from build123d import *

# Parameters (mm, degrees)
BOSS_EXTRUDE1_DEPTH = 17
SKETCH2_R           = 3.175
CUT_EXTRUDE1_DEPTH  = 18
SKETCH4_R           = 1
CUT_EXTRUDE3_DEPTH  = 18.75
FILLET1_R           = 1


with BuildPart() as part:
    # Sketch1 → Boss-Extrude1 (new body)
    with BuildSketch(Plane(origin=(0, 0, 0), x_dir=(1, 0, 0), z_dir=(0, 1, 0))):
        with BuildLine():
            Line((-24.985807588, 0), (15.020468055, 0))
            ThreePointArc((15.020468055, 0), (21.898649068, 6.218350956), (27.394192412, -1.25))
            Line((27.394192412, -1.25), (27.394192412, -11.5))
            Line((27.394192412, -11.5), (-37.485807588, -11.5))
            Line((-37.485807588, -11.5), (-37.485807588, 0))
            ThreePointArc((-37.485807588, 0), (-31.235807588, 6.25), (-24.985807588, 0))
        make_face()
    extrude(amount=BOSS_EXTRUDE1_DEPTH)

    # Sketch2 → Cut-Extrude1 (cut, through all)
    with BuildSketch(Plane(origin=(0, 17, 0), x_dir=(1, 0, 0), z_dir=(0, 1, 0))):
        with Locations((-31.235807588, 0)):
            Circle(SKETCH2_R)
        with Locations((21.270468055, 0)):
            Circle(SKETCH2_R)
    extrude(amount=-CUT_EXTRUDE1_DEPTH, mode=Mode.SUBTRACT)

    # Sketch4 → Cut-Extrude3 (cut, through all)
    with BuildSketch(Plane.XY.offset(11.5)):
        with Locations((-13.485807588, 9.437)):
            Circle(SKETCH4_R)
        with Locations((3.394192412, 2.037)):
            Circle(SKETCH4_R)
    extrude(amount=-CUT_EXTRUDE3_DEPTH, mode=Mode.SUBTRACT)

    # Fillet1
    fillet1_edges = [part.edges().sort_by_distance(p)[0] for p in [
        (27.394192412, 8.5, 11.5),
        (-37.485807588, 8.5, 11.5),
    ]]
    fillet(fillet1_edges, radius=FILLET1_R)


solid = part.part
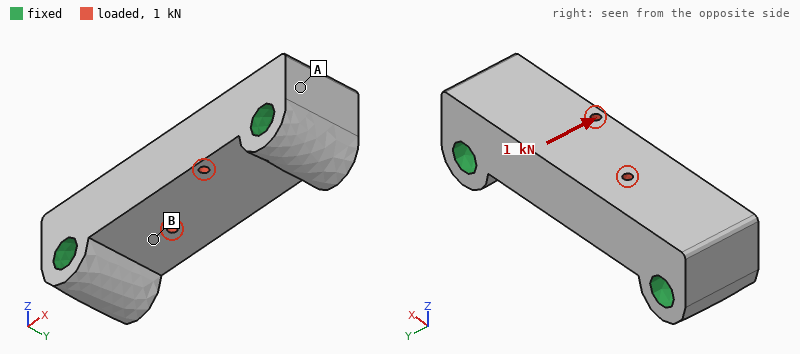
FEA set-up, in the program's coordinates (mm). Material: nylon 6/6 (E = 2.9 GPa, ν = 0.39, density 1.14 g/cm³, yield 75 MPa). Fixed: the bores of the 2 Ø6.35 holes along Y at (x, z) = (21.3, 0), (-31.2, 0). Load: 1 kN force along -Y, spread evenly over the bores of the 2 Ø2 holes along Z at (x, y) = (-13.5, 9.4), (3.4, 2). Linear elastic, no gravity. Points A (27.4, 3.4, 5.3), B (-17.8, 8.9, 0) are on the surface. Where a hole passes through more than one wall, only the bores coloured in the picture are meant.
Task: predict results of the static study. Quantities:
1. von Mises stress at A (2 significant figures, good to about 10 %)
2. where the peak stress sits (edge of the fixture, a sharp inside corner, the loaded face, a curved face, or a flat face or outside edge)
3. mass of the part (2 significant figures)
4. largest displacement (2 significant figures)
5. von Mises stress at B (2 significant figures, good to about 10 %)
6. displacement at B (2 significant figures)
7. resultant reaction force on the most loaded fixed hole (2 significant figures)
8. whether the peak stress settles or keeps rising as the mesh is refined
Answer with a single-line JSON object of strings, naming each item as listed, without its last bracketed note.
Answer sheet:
{"von Mises stress at A": "2.0 MPa", "where the peak stress sits": "edge of the fixture", "mass of the part": "16 g", "largest displacement": "0.10 mm", "von Mises stress at B": "7.2 MPa", "displacement at B": "0.059 mm", "resultant reaction force on the most loaded fixed hole": "500 N", "whether the peak stress settles or keeps rising as the mesh is refined": "keeps rising"}
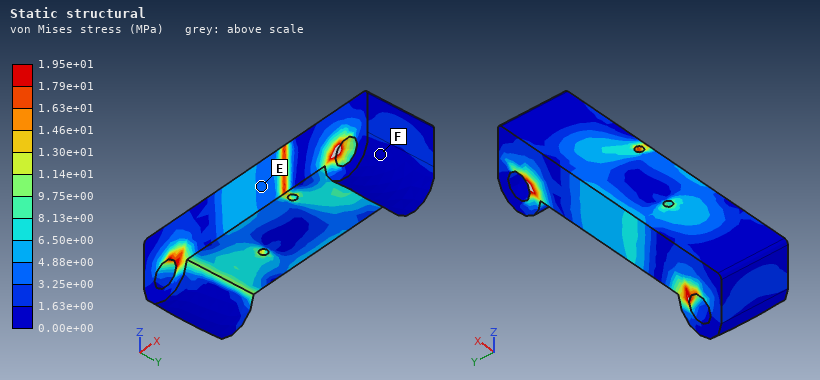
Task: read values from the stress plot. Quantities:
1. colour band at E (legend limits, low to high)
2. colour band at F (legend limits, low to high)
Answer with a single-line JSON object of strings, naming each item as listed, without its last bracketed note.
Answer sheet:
{"colour band at E": "3.25e+00 to 4.88e+00 MPa", "colour band at F": "0.00e+00 to 1.63e+00 MPa"}
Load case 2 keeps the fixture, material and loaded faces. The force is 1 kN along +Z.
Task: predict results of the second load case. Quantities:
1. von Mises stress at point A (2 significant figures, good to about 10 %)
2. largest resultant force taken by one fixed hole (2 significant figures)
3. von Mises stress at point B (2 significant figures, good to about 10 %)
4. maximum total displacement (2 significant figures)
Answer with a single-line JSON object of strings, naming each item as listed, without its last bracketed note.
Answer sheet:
{"von Mises stress at point A": "2.9 MPa", "largest resultant force taken by one fixed hole": "620 N", "von Mises stress at point B": "3.8 MPa", "maximum total displacement": "0.18 mm"}
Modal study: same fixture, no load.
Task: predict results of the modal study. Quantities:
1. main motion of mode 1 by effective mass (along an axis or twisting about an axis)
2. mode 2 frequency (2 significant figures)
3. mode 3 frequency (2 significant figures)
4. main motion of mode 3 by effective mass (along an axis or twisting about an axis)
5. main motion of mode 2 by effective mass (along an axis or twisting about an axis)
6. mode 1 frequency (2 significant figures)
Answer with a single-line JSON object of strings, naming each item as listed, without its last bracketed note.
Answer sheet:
{"main motion of mode 1 by effective mass": "along Z", "mode 2 frequency": "6500 Hz", "mode 3 frequency": "8700 Hz", "main motion of mode 3 by effective mass": "twisting about X", "main motion of mode 2 by effective mass": "along Y", "mode 1 frequency": "5700 Hz"}
